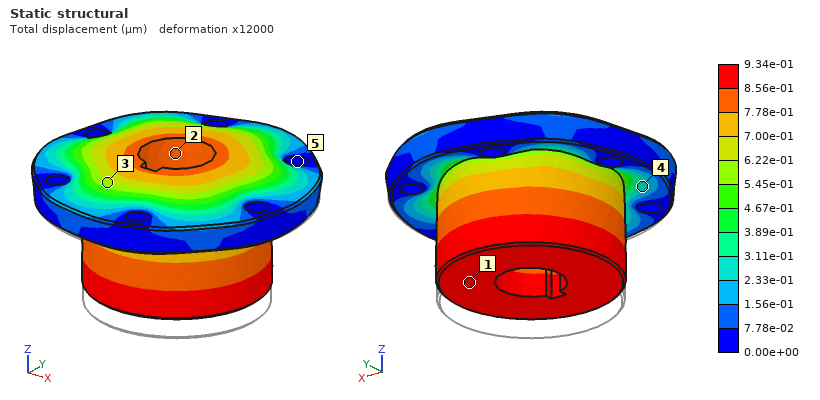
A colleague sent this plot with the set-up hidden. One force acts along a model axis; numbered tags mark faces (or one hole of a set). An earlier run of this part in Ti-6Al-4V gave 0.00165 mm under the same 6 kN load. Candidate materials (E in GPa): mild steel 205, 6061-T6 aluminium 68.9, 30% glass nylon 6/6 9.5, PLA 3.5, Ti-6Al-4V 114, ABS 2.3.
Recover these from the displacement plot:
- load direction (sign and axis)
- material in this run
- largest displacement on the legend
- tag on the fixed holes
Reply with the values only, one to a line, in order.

+Z
mild steel
9.34e-01 µm
5
